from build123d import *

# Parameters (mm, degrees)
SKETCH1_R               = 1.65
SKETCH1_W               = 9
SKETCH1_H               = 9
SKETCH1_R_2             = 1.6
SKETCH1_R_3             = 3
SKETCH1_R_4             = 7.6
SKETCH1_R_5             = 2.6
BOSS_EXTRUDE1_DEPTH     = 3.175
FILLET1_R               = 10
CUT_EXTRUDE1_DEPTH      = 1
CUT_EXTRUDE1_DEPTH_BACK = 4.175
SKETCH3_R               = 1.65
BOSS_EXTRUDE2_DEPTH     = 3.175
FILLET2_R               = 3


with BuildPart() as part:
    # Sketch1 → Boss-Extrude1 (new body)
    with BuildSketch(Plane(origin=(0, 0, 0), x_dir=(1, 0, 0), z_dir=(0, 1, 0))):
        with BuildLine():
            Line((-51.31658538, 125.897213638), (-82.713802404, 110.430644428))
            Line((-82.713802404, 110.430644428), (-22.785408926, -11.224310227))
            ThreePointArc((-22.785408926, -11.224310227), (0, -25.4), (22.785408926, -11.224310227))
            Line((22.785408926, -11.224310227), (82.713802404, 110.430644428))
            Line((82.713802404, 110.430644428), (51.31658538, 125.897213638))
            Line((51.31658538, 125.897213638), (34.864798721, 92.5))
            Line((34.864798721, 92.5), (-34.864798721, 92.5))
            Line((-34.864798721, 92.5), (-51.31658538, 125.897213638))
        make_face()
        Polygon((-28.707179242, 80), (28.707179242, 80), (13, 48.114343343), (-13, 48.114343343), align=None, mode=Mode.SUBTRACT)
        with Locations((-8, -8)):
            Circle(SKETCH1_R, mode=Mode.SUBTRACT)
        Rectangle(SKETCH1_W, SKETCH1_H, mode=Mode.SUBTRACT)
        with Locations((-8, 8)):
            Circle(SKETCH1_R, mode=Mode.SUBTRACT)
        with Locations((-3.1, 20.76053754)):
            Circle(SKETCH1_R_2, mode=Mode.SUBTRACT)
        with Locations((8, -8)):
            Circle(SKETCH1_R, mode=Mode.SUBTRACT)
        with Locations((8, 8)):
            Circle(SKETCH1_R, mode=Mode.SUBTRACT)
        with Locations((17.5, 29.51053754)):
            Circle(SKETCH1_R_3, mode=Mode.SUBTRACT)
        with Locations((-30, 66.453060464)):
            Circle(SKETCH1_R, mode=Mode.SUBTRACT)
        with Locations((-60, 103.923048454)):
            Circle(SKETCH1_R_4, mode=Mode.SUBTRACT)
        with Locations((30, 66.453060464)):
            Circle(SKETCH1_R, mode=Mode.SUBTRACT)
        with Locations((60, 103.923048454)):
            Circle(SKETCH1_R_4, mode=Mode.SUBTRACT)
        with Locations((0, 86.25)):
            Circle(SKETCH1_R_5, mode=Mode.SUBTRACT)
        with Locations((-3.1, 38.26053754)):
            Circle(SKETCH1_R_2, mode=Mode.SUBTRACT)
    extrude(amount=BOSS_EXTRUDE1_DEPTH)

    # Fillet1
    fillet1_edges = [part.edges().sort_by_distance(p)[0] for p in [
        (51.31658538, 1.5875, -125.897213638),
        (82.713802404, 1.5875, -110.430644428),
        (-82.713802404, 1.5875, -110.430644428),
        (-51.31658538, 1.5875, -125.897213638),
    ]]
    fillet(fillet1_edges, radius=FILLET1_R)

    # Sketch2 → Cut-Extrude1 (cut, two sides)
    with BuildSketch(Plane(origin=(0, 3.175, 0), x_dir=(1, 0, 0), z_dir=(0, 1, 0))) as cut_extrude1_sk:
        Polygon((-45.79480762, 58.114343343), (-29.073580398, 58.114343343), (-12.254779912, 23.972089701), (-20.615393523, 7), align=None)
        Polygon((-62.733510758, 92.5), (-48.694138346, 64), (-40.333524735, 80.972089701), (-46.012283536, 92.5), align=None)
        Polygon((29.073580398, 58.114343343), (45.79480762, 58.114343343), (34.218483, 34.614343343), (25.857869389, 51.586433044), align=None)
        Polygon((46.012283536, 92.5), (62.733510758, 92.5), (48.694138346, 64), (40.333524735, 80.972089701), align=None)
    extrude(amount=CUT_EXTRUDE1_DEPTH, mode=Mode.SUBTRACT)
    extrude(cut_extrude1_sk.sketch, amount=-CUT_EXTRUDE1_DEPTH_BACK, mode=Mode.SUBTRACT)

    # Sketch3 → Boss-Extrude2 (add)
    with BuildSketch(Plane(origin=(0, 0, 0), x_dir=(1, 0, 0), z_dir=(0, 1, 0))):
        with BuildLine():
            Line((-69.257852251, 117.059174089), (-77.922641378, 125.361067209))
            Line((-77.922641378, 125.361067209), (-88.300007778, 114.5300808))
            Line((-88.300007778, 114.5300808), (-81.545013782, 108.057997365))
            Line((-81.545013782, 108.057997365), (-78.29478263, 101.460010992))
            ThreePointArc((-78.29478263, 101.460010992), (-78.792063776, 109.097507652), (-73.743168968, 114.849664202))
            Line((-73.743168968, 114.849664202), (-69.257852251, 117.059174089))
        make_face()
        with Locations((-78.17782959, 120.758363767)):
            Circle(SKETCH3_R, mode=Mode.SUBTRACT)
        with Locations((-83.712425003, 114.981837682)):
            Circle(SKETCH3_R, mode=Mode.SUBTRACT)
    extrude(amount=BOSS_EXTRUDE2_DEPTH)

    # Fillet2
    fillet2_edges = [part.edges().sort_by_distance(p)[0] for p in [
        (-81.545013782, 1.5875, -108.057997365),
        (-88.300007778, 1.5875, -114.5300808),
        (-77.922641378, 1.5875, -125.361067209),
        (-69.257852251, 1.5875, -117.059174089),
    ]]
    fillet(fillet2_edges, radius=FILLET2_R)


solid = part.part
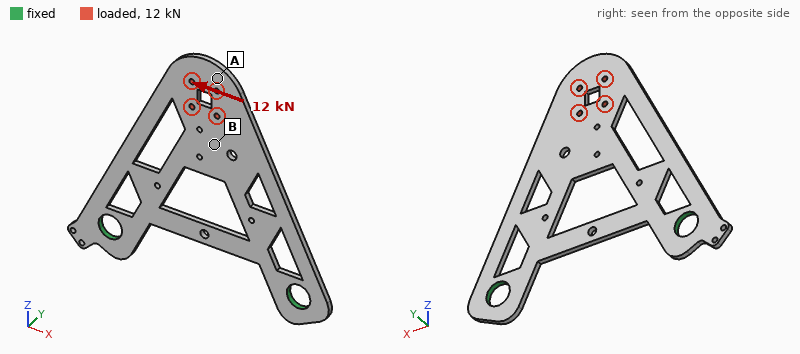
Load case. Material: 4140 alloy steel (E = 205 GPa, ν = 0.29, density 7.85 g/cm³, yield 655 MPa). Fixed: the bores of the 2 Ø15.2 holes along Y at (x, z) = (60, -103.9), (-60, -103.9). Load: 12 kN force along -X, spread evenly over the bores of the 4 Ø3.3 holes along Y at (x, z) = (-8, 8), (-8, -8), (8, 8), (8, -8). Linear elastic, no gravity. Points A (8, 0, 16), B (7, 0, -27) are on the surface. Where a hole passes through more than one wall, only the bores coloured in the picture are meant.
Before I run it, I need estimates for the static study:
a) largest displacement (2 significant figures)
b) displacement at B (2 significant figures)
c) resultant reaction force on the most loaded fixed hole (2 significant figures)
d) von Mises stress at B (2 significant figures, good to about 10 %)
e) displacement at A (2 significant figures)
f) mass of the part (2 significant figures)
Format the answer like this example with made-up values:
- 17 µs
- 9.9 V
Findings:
- 0.20 mm
- 0.13 mm
- 11 kN
- 130 MPa
- 0.19 mm
- 220 g
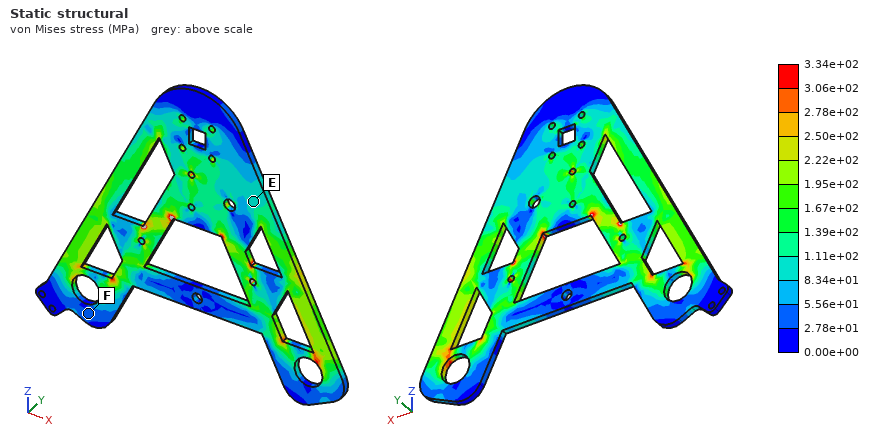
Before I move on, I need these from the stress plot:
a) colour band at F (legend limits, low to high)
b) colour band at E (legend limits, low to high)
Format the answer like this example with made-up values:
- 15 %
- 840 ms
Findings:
- 2.78e+01 to 5.56e+01 MPa
- 8.34e+01 to 1.11e+02 MPa
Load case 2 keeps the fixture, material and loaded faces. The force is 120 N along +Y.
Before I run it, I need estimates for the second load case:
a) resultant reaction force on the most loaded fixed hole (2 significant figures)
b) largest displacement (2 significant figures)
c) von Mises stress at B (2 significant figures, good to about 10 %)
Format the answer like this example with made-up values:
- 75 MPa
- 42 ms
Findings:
- 61 N
- 2.3 mm
- 40 MPa
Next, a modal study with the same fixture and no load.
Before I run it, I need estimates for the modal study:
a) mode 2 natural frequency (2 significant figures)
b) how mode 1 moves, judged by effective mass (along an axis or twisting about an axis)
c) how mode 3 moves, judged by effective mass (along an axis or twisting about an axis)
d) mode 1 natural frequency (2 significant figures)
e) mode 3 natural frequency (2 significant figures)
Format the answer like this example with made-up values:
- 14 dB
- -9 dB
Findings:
- 750 Hz
- along Y
- along Y
- 160 Hz
- 870 Hz
